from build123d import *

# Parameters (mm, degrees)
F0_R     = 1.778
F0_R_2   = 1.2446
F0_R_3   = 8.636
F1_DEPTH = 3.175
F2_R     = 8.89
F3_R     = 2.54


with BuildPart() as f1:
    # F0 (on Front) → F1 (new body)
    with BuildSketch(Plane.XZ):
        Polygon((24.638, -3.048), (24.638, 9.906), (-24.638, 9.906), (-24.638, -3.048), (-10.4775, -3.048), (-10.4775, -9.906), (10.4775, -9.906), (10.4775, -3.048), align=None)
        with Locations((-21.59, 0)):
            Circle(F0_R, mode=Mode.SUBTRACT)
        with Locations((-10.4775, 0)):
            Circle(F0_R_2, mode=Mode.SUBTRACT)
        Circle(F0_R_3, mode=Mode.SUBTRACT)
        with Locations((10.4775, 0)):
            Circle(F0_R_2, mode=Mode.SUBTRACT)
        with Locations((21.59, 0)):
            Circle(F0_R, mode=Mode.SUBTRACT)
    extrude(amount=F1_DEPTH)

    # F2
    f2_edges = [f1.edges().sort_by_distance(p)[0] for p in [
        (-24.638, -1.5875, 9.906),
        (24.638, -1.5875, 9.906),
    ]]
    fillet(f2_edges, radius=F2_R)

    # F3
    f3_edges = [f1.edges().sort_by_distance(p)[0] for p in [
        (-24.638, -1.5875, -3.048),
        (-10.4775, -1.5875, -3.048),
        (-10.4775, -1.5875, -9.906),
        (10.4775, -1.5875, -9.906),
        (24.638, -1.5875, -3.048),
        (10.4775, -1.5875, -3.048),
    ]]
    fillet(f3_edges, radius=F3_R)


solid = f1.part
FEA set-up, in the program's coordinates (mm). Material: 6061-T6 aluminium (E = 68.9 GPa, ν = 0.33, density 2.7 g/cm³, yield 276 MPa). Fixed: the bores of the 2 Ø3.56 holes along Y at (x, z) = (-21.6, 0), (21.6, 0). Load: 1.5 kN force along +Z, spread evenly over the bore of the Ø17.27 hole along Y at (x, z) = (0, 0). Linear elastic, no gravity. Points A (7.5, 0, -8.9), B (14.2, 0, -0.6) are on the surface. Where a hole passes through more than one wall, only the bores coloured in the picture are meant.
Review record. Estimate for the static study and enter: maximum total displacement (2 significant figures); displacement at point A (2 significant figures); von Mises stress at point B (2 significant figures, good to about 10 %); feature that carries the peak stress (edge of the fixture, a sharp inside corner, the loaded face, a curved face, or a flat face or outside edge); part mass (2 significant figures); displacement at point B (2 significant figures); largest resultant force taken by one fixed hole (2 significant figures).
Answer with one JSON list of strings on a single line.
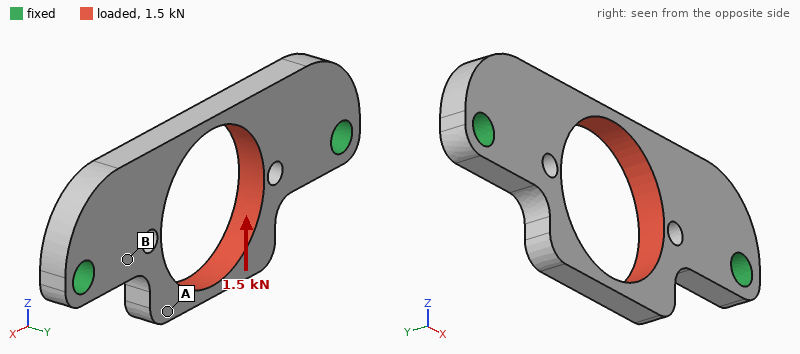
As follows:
["39 µm", "30 µm", "49 MPa", "edge of the fixture", "4.1 g", "16 µm", "810 N"]
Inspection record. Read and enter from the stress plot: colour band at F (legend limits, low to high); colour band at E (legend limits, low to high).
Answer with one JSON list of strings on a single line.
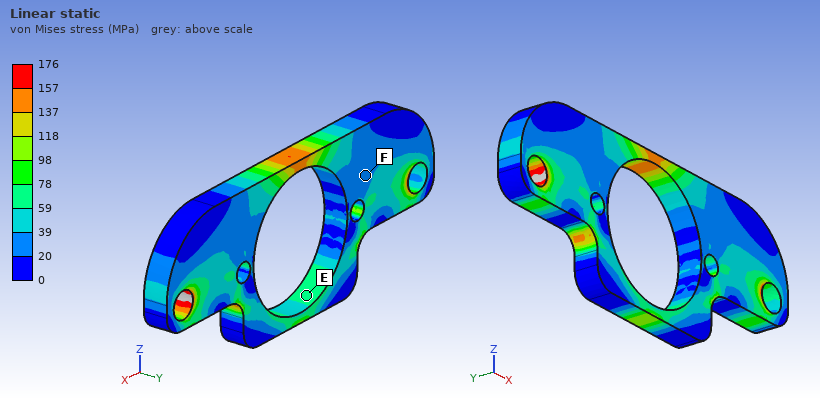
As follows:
["20 to 39 MPa", "59 to 78 MPa"]
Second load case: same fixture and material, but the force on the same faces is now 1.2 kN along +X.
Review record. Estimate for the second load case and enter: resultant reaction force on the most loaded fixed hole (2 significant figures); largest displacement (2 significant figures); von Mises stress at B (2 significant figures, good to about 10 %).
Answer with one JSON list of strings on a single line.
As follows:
["600 N", "26 µm", "25 MPa"]
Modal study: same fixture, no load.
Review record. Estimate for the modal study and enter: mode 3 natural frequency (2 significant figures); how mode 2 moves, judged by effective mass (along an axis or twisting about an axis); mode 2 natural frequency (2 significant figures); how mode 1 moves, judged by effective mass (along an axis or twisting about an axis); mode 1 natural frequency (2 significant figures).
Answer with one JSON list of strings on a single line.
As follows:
["17 kHz", "along Y", "10000 Hz", "along Y", "8300 Hz"]
